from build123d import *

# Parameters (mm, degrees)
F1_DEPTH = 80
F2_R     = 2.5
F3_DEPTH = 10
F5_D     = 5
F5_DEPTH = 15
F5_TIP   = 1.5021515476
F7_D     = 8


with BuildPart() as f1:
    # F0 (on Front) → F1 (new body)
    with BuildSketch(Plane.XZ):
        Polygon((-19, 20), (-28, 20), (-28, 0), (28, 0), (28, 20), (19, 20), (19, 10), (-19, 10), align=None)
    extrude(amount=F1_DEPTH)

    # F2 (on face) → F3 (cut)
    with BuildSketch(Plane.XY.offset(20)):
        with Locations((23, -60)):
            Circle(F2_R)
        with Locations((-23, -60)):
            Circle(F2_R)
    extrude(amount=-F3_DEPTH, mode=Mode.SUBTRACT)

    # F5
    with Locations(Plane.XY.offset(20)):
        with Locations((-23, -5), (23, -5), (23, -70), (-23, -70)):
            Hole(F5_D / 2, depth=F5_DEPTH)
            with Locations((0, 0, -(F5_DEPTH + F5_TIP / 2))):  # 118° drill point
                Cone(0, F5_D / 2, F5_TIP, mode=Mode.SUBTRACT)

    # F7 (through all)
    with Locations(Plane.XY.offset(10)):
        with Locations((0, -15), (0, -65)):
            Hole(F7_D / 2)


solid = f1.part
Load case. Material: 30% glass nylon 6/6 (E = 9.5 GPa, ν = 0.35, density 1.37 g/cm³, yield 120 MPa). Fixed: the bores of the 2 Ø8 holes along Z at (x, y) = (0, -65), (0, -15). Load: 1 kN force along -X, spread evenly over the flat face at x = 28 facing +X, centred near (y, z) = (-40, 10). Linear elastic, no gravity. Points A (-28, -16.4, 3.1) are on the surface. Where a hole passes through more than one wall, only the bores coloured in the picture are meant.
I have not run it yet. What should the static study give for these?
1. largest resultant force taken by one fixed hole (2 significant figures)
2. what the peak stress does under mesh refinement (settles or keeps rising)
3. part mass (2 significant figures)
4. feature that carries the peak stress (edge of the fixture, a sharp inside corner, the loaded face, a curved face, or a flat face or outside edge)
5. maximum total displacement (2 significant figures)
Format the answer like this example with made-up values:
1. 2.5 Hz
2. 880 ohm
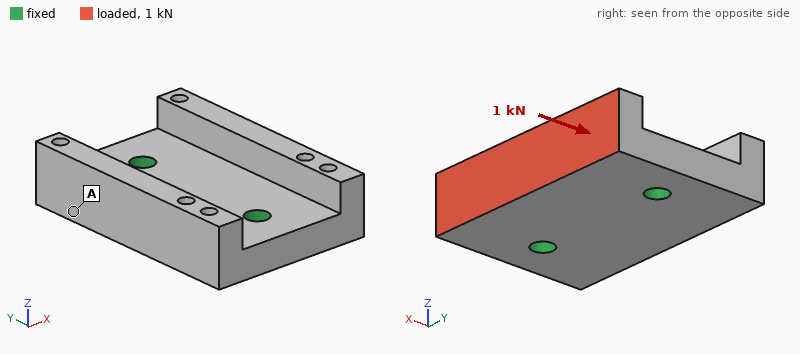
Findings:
1. 500 N
2. keeps rising
3. 78 g
4. edge of the fixture
5. 48 µm
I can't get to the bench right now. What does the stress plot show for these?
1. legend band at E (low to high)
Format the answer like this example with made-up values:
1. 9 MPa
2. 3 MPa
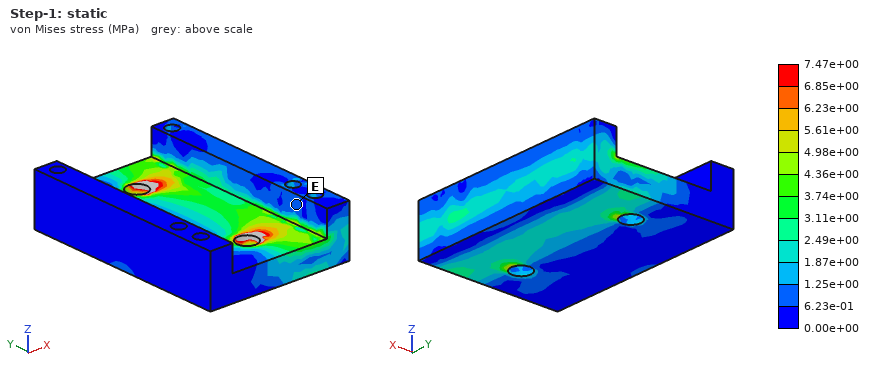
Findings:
1. 6.23e-01 to 1.25e+00 MPa
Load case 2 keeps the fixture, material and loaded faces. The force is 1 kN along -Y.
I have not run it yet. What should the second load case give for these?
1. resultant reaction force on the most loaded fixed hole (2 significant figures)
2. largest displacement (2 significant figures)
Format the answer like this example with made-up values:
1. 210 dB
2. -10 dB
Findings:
1. 710 N
2. 27 µm
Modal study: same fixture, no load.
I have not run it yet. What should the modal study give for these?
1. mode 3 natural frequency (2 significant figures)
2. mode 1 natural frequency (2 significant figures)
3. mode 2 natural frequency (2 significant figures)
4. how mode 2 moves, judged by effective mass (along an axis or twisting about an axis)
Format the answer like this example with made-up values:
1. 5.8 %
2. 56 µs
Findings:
1. 4700 Hz
2. 3000 Hz
3. 3900 Hz
4. along Z
